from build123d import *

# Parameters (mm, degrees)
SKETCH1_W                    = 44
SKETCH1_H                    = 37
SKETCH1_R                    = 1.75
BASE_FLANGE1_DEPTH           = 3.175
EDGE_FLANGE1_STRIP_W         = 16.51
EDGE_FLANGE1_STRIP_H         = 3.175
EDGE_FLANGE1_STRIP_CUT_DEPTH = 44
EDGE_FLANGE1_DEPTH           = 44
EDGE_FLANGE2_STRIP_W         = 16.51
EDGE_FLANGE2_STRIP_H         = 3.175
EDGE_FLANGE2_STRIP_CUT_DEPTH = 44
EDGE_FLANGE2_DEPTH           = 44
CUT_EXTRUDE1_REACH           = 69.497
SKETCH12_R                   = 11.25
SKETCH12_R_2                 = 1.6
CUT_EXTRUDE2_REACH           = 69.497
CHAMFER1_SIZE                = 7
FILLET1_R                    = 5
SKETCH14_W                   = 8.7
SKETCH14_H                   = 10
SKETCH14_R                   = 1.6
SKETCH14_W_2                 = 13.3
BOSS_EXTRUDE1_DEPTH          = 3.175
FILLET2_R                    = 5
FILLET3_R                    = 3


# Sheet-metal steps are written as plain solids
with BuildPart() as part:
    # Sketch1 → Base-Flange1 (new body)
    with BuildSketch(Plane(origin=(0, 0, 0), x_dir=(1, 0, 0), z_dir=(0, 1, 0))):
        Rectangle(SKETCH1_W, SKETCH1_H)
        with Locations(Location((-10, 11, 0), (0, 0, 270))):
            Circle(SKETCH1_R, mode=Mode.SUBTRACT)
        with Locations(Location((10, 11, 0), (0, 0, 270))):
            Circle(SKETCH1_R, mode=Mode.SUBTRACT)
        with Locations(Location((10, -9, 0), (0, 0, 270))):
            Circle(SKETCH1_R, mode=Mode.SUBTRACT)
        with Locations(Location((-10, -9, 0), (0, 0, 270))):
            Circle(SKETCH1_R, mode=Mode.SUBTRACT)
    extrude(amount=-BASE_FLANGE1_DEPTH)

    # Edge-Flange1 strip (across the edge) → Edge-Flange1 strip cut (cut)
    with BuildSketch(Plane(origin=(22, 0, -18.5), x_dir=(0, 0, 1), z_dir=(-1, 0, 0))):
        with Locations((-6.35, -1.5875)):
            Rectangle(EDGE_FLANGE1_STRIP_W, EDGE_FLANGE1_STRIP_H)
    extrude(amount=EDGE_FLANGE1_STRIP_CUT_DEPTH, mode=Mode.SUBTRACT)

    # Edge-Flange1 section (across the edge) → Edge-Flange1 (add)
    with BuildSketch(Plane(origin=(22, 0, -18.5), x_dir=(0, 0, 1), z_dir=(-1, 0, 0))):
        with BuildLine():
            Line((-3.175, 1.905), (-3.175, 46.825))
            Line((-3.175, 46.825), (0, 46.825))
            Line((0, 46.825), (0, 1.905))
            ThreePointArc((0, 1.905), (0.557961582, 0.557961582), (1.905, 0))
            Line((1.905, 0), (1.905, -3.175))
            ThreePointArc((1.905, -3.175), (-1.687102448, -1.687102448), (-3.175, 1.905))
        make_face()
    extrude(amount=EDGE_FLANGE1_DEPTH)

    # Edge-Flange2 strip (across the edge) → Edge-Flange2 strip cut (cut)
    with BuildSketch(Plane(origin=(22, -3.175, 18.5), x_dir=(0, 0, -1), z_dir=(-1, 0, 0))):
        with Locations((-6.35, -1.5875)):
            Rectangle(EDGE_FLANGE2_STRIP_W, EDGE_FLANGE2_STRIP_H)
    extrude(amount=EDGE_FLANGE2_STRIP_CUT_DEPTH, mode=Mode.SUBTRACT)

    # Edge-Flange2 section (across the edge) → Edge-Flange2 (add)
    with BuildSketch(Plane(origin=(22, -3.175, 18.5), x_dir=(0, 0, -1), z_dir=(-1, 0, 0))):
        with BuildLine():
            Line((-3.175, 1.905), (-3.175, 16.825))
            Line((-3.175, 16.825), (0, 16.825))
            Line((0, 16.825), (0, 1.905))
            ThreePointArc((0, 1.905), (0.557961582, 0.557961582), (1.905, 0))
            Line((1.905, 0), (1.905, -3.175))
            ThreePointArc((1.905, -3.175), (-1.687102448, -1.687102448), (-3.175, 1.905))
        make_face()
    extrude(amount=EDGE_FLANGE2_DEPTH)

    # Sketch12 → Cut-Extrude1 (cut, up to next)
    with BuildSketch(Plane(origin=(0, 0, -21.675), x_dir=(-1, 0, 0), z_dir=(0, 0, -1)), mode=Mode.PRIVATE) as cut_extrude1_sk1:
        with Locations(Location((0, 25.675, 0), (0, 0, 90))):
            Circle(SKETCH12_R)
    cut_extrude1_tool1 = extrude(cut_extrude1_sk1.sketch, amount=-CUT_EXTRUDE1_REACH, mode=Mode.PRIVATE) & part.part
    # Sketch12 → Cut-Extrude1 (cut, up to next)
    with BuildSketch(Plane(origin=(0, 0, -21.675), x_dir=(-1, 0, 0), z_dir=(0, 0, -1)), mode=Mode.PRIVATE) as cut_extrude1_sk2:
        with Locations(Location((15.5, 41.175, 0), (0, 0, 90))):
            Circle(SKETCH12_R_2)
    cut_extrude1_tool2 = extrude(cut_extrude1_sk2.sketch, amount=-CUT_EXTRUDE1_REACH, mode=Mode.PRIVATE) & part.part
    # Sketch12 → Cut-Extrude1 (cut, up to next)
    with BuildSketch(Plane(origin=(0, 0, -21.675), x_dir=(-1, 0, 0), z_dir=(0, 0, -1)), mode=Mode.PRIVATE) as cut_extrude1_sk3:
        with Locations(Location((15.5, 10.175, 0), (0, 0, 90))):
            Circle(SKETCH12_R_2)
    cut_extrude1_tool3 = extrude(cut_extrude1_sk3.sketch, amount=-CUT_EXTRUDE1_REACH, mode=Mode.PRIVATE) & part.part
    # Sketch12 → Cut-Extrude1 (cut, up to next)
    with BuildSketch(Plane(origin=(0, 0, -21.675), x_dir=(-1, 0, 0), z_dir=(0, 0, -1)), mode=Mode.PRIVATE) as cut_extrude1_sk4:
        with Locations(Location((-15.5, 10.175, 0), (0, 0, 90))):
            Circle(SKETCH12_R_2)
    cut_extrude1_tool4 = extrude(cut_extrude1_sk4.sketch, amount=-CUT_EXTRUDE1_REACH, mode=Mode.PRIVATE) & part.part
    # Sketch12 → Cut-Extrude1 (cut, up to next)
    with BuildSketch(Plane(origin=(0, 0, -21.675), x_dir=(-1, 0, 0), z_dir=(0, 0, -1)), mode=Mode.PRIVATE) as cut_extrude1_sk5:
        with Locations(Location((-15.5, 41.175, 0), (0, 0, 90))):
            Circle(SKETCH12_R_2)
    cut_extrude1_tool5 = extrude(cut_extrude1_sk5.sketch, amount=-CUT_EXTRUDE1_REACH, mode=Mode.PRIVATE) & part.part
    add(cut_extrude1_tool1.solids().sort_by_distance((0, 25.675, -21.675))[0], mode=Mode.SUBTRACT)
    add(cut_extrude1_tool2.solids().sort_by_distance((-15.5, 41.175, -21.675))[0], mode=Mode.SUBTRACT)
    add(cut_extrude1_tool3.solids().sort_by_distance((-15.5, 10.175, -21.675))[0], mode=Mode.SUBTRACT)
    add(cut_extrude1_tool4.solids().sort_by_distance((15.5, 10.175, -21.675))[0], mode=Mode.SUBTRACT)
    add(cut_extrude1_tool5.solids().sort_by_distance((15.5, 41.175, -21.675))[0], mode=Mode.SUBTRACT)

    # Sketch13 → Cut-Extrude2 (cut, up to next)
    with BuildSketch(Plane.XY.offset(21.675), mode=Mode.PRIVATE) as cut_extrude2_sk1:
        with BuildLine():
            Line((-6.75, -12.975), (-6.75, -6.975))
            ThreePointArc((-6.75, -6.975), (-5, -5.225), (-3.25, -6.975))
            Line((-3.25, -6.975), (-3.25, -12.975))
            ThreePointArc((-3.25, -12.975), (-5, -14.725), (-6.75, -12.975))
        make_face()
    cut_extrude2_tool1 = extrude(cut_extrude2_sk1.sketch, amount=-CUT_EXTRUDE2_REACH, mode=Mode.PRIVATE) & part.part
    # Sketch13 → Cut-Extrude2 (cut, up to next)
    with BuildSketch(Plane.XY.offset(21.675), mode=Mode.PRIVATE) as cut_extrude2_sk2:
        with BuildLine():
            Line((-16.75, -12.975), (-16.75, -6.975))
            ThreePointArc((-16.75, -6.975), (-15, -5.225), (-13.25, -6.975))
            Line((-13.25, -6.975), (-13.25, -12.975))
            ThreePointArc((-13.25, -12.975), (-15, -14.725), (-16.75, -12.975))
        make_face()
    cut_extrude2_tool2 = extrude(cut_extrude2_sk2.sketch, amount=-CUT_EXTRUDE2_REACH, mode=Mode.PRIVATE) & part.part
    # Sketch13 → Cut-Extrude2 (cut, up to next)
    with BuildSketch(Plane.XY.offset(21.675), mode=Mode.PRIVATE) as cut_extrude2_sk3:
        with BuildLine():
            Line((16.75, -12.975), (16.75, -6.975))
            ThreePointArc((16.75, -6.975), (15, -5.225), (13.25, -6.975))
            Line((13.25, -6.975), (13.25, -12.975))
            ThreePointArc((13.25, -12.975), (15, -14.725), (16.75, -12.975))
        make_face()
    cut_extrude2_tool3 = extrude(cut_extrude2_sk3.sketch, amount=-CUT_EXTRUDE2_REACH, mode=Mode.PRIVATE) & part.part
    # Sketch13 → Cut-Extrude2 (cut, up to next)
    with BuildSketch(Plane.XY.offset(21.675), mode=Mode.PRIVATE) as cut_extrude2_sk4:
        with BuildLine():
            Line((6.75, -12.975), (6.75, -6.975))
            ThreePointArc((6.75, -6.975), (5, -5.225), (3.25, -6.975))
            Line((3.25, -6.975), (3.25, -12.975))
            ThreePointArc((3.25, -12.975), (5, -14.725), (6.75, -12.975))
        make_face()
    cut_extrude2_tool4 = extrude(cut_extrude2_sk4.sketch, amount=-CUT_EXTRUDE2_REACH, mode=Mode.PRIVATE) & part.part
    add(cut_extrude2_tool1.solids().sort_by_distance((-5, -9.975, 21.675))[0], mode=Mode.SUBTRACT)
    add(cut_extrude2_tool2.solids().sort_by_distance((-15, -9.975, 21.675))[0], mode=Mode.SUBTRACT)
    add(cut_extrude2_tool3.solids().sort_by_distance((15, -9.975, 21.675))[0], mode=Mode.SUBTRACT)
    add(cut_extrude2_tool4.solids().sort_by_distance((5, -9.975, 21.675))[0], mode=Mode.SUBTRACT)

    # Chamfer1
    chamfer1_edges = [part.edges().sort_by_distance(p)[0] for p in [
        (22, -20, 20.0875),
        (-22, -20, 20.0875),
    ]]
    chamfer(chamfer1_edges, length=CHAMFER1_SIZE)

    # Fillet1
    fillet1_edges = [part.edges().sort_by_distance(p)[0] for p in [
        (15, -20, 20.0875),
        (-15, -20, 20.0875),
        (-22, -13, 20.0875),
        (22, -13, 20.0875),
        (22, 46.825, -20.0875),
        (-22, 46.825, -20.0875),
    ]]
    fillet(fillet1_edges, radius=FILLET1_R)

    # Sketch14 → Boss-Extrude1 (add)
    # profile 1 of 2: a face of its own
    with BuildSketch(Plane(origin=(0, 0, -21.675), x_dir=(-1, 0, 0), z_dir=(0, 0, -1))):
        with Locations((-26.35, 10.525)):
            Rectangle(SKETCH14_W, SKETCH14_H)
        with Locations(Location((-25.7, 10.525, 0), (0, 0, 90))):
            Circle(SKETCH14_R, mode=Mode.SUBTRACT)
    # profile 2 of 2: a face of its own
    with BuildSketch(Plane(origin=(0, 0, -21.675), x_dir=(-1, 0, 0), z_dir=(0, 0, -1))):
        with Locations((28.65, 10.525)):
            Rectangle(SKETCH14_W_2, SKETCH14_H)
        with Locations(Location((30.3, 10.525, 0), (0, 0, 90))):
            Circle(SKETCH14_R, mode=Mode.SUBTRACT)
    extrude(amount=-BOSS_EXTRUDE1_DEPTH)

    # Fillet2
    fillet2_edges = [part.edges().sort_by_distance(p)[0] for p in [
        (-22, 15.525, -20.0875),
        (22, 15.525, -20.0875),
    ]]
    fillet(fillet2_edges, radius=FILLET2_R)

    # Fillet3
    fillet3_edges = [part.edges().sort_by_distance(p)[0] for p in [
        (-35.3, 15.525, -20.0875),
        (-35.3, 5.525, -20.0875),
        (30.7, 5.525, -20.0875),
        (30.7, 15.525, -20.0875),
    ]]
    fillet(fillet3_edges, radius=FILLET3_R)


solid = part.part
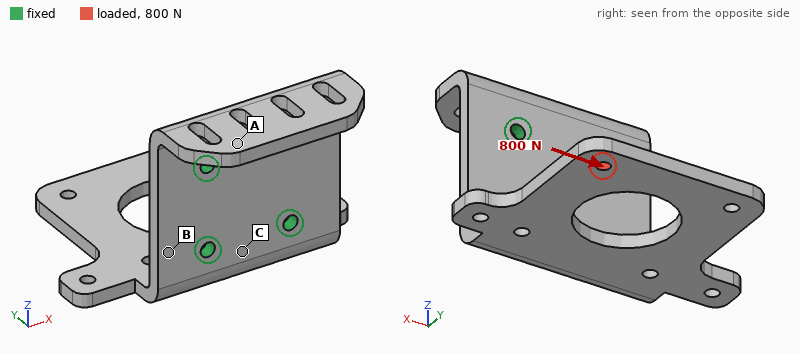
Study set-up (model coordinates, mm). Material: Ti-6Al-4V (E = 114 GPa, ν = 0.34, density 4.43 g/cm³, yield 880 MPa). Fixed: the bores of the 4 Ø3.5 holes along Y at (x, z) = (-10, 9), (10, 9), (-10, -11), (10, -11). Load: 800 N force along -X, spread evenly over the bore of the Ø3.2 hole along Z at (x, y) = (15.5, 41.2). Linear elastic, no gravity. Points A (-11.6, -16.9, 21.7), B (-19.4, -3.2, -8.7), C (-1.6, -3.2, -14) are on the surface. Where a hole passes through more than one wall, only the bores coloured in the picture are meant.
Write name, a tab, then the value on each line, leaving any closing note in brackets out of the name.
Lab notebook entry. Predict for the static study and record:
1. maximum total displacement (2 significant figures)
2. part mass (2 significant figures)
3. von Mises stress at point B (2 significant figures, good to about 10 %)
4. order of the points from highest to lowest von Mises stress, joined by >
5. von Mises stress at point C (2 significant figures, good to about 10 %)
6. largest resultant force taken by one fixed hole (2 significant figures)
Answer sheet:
maximum total displacement	0.24 mm
part mass	58 g
von Mises stress at point B	89 MPa
order of the points from highest to lowest von Mises stress, joined by >	B > C > A
von Mises stress at point C	59 MPa
largest resultant force taken by one fixed hole	1.6 kN
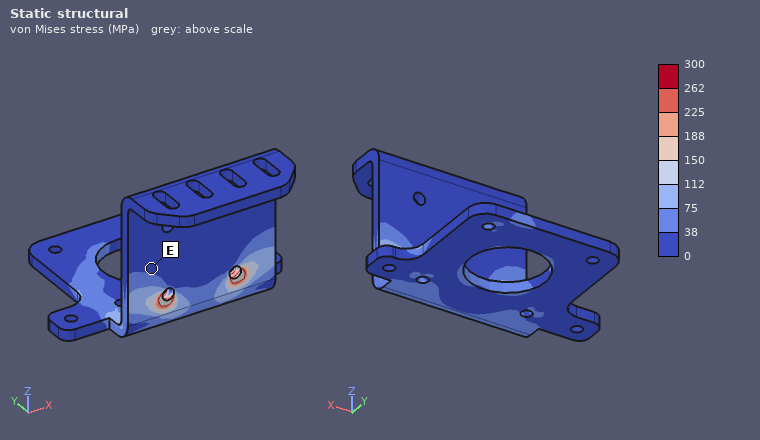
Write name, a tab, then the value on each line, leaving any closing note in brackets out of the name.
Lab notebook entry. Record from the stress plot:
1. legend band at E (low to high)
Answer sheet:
legend band at E	0 to 38 MPa
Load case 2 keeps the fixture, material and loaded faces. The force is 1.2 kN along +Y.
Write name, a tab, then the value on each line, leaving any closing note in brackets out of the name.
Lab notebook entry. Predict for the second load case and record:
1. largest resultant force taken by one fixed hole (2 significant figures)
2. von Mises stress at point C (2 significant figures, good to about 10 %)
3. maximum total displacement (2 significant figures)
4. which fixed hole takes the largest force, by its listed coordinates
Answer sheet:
largest resultant force taken by one fixed hole	1.5 kN
von Mises stress at point C	62 MPa
maximum total displacement	0.27 mm
which fixed hole takes the largest force, by its listed coordinates	(10, -11)
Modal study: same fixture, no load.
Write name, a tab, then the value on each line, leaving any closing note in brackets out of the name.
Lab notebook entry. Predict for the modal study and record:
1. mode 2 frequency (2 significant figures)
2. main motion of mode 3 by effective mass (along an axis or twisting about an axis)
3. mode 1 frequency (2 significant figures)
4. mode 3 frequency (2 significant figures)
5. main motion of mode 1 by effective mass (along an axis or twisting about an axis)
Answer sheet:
mode 2 frequency	2200 Hz
main motion of mode 3 by effective mass	along X
mode 1 frequency	930 Hz
mode 3 frequency	3300 Hz
main motion of mode 1 by effective mass	along Z
